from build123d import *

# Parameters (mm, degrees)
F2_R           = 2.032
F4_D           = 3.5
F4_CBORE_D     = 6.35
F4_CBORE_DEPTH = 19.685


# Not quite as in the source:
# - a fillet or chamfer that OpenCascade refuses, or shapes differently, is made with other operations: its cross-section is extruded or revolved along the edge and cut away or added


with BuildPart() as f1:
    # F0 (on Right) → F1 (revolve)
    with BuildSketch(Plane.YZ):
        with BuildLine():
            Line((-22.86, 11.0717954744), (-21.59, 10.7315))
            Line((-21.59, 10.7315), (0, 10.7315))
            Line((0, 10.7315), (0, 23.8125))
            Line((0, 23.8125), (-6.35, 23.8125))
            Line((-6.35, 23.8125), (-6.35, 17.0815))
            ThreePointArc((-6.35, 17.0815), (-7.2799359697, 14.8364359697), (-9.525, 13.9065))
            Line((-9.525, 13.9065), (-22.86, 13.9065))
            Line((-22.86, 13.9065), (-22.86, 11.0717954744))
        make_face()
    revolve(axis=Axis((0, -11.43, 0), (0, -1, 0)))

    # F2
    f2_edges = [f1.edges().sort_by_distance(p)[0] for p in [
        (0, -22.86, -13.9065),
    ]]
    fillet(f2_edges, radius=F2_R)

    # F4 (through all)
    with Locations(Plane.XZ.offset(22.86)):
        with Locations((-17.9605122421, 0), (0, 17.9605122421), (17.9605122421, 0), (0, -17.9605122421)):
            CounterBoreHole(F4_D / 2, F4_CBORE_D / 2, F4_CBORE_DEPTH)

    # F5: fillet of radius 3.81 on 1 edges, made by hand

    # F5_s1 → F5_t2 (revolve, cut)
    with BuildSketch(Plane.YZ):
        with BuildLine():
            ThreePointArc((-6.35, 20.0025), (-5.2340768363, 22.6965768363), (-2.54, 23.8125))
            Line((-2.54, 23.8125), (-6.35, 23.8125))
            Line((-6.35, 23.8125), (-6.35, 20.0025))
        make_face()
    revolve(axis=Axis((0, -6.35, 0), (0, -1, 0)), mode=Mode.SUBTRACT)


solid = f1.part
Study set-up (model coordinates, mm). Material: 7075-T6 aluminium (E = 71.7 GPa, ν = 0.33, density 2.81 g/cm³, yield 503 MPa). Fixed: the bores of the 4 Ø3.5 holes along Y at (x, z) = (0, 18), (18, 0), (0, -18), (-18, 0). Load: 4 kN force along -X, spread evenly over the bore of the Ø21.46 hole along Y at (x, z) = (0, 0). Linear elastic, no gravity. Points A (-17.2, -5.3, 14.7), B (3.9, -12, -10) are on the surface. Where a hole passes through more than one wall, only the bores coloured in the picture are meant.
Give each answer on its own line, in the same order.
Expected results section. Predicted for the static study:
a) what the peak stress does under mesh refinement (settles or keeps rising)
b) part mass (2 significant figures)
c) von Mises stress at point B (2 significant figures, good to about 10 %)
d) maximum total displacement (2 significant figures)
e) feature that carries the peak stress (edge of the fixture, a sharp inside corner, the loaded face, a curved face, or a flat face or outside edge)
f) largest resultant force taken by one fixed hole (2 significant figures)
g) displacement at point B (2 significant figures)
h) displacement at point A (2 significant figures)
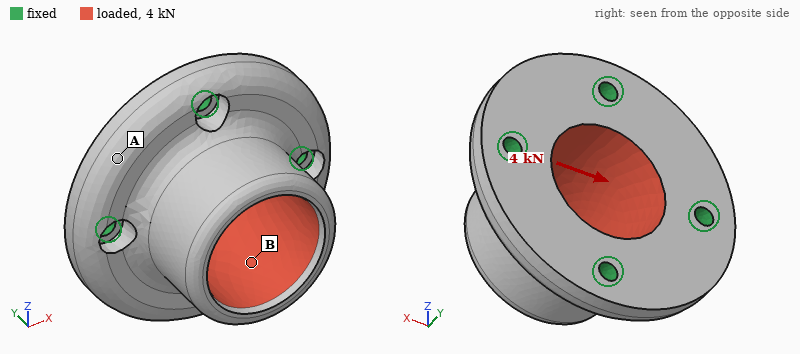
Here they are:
keeps rising
34 g
24 MPa
16 µm
edge of the fixture
1.5 kN
9.2 µm
7.1 µm
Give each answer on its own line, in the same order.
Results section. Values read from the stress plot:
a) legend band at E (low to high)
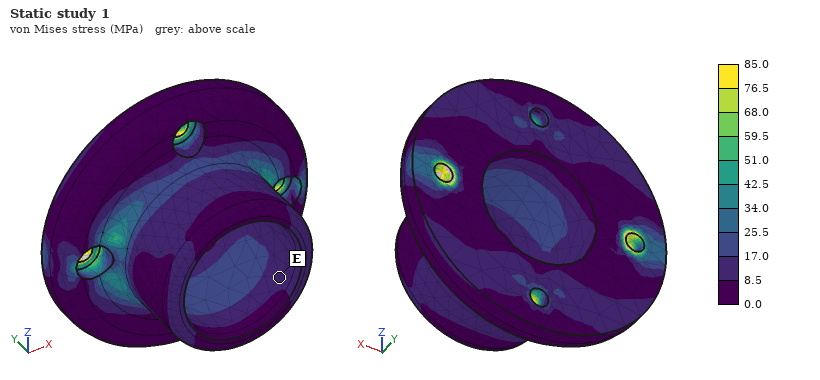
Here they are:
8.5 to 17.0 MPa
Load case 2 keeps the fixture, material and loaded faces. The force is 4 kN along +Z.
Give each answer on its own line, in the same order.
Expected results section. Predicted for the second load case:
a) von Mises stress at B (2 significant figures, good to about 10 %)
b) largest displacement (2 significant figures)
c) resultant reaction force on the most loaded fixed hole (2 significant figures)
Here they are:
17 MPa
16 µm
1.5 kN
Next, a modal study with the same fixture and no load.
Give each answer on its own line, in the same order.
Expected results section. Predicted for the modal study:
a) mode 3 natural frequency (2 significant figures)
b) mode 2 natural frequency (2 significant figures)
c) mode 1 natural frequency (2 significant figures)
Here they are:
19 kHz
19 kHz
17 kHz
